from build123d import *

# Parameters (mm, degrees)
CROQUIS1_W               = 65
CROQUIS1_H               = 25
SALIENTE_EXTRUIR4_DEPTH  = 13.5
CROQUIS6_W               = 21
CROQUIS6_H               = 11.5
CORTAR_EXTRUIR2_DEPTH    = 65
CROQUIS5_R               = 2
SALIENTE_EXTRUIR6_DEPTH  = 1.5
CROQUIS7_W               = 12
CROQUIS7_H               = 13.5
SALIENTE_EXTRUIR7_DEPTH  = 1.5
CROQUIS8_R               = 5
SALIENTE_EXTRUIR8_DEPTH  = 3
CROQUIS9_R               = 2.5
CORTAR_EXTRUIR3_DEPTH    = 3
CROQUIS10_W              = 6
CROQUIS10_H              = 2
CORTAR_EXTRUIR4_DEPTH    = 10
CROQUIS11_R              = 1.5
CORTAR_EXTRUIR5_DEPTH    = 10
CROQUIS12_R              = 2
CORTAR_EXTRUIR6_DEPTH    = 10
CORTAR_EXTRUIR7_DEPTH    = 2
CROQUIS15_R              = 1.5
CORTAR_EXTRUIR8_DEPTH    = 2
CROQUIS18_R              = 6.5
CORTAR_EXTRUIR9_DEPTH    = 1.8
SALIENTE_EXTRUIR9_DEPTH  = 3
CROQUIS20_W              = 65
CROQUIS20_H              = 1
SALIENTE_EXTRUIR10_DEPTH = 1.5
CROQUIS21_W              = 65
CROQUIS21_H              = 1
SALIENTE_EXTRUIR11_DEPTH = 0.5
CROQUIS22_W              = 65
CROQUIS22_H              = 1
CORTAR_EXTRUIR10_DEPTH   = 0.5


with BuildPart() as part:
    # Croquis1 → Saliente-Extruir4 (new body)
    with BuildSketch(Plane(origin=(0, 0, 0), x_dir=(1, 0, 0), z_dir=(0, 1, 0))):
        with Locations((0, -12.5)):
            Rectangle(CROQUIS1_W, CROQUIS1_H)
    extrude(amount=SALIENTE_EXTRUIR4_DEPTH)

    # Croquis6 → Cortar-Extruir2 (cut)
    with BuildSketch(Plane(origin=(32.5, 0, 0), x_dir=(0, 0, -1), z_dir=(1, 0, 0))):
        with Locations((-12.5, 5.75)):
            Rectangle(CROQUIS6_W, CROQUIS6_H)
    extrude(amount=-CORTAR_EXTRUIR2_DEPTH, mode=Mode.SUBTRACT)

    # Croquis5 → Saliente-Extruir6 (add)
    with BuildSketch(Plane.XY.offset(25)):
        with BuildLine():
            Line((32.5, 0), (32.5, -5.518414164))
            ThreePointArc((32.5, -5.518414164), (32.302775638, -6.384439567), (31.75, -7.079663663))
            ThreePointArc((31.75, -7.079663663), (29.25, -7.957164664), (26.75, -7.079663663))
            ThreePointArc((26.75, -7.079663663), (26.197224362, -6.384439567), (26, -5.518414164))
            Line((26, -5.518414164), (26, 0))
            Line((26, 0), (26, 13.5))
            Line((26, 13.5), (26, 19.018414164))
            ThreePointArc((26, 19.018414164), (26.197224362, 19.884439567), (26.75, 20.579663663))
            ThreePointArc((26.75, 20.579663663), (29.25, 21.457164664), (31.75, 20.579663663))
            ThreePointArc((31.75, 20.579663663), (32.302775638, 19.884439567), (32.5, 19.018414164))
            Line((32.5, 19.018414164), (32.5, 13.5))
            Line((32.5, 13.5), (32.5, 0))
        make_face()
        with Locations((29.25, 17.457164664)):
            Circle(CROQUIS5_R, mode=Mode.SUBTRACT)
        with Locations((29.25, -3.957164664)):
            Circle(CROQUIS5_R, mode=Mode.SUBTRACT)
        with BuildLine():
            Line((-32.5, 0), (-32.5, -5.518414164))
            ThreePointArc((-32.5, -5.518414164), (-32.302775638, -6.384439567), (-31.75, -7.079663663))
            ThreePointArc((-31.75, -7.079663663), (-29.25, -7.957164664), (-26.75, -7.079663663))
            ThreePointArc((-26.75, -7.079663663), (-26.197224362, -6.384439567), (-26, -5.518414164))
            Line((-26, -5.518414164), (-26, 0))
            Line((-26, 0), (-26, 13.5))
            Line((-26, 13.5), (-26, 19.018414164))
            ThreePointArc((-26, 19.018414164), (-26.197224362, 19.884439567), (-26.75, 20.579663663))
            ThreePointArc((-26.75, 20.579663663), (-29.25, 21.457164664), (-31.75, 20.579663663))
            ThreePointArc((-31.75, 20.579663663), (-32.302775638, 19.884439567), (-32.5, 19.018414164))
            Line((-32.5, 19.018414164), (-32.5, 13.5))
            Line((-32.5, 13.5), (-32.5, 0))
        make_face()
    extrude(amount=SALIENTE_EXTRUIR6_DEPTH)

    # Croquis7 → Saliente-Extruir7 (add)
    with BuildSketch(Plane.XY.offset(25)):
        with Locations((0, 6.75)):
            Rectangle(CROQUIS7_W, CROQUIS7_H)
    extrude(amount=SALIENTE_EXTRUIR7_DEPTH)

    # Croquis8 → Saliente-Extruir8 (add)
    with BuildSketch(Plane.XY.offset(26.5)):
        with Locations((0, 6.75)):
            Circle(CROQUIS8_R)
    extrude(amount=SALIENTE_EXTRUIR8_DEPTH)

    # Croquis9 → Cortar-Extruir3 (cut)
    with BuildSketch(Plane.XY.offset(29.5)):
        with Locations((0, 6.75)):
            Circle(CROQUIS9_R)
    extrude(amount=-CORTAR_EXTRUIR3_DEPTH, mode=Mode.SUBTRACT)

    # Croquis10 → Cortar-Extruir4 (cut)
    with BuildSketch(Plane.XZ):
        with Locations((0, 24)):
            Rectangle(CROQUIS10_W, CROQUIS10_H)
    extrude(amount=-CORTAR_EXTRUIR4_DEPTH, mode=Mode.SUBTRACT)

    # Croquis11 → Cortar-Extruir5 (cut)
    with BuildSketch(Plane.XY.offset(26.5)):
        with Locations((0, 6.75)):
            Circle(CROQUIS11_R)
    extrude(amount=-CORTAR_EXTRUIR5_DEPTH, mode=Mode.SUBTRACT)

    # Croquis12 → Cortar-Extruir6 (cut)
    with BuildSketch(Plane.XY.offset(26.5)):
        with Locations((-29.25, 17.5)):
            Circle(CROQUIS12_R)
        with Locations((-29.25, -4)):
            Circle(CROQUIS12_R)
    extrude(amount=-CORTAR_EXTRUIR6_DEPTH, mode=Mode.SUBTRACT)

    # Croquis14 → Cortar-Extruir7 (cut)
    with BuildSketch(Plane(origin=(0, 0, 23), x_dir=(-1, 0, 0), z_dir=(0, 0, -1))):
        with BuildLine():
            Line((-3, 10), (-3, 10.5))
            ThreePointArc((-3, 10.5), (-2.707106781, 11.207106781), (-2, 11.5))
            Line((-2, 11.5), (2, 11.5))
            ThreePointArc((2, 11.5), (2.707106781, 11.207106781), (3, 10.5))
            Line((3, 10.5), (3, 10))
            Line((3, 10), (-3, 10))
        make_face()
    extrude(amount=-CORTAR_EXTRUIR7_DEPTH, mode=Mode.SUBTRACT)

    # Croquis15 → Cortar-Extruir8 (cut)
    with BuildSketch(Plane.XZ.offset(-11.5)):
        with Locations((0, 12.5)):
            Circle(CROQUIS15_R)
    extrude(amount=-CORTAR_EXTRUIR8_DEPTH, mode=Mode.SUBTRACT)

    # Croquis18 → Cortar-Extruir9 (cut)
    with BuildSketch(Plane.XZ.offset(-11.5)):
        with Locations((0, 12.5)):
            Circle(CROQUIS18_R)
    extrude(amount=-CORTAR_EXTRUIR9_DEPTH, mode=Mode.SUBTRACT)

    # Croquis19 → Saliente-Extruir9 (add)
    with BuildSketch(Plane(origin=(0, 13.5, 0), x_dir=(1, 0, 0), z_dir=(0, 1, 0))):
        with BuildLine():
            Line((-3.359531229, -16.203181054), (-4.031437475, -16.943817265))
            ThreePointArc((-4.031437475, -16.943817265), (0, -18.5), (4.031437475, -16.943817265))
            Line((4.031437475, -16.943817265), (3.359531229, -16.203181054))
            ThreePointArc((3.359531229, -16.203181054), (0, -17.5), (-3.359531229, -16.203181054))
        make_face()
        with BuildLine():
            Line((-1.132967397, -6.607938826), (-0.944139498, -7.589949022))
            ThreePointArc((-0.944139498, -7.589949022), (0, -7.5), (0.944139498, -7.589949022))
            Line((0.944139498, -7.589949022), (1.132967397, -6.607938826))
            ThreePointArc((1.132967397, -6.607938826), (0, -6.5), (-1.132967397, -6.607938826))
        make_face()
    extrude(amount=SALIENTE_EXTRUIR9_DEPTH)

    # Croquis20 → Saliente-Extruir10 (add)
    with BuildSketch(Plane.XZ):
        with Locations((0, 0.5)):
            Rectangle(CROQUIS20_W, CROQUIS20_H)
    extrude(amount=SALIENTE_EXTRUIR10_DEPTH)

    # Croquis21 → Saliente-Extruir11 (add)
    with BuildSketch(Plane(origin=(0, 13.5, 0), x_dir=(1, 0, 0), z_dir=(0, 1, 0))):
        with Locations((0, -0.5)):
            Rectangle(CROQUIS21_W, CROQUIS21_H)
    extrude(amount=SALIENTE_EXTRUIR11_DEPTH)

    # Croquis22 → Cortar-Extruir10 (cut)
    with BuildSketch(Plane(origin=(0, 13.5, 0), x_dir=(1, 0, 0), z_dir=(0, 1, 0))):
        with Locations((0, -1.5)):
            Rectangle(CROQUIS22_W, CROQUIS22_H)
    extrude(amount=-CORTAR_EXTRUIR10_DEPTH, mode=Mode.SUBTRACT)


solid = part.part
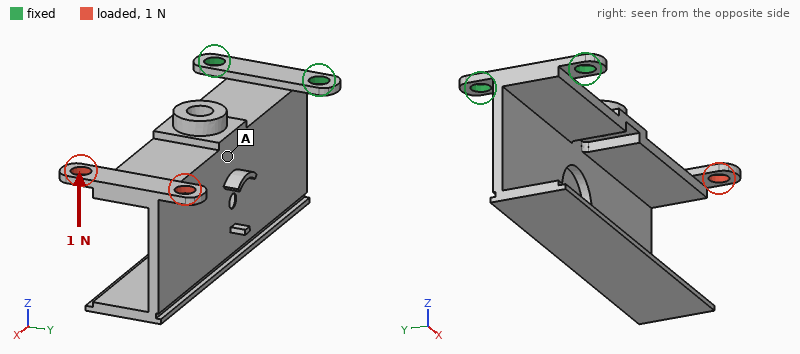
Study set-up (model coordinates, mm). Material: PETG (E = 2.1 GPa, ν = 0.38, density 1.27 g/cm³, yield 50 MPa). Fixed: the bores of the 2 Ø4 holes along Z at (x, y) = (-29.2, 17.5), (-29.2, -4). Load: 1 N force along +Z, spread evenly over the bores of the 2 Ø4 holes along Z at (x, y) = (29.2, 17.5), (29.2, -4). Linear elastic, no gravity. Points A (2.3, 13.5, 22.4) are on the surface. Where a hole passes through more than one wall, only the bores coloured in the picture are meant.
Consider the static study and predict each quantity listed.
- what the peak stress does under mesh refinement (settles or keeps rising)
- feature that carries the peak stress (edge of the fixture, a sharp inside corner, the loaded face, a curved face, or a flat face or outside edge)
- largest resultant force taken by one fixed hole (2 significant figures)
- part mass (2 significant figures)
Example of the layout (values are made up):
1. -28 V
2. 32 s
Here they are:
1. keeps rising
2. edge of the fixture
3. 1.3 N
4. 8.7 g
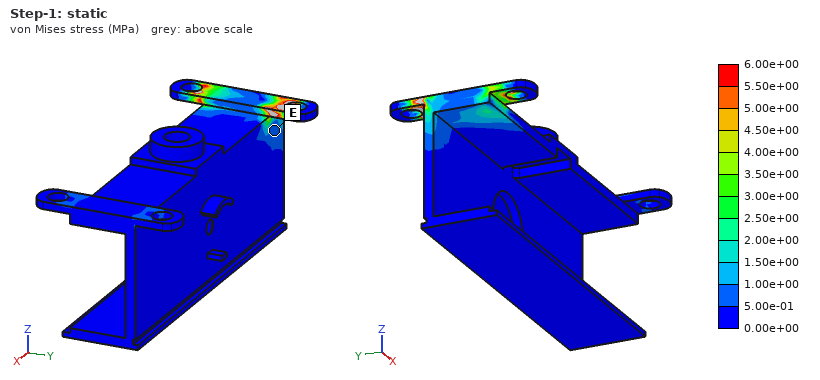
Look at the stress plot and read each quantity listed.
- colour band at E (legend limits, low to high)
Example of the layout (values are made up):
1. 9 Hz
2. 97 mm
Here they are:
1. 5.00e-01 to 1.00e+00 MPa
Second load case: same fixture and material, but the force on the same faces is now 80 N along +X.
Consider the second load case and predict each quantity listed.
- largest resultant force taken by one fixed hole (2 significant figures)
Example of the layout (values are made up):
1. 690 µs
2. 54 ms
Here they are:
1. 41 N
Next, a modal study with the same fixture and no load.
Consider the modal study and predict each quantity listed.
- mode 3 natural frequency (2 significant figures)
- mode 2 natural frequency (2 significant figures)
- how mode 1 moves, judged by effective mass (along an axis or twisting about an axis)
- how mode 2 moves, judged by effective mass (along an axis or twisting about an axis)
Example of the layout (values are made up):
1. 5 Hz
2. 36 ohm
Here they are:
1. 410 Hz
2. 180 Hz
3. along Z
4. along Y
